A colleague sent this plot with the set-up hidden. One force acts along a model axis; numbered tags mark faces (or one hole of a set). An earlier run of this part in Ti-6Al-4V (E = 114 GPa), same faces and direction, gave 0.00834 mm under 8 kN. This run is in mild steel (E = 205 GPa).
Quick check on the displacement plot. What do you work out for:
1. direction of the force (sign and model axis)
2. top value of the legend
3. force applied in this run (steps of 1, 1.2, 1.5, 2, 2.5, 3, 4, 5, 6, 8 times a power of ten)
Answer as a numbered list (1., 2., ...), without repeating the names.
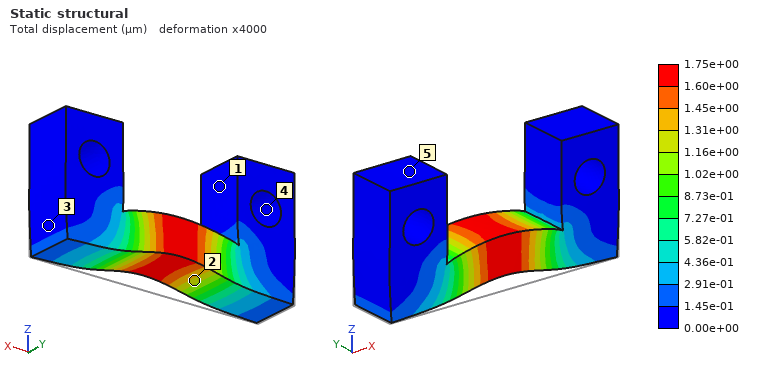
1. +Z
2. 1.75e+00 µm
3. 3 kN
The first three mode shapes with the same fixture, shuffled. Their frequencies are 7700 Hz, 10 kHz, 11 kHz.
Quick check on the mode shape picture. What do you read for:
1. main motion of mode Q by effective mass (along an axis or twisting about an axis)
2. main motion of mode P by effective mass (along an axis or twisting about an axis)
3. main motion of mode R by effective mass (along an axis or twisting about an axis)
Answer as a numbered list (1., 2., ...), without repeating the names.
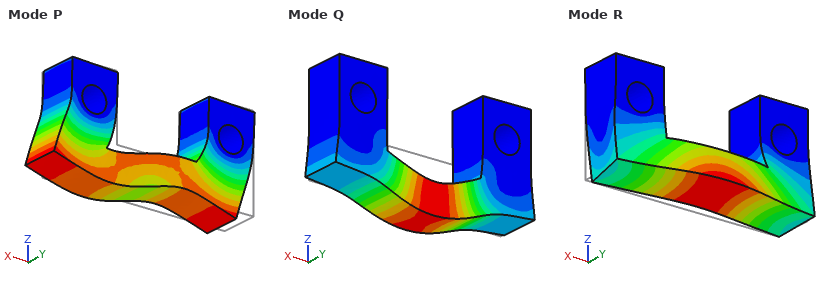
1. along Z
2. along X
3. along Y
